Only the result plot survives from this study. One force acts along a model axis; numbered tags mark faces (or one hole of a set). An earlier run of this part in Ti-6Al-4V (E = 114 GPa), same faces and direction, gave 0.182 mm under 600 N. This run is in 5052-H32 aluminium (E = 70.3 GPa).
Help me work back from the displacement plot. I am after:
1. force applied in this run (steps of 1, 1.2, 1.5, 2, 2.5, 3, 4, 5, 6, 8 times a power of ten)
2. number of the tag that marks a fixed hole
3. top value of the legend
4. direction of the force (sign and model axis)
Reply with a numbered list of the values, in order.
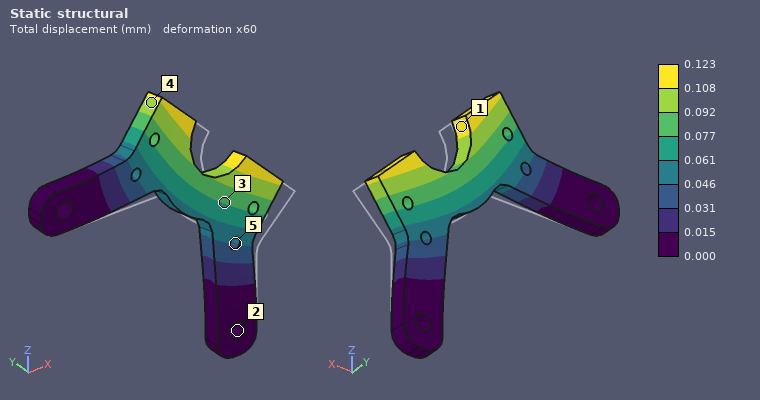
1. 250 N
2. 2
3. 0.123 mm
4. +Y
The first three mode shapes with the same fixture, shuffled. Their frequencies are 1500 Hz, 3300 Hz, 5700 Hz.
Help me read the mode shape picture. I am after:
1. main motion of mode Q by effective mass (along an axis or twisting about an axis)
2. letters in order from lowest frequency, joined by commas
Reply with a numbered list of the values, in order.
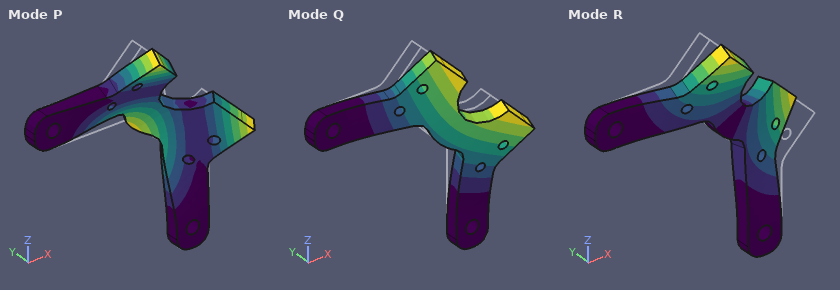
1. along Y
2. Q, R, P
